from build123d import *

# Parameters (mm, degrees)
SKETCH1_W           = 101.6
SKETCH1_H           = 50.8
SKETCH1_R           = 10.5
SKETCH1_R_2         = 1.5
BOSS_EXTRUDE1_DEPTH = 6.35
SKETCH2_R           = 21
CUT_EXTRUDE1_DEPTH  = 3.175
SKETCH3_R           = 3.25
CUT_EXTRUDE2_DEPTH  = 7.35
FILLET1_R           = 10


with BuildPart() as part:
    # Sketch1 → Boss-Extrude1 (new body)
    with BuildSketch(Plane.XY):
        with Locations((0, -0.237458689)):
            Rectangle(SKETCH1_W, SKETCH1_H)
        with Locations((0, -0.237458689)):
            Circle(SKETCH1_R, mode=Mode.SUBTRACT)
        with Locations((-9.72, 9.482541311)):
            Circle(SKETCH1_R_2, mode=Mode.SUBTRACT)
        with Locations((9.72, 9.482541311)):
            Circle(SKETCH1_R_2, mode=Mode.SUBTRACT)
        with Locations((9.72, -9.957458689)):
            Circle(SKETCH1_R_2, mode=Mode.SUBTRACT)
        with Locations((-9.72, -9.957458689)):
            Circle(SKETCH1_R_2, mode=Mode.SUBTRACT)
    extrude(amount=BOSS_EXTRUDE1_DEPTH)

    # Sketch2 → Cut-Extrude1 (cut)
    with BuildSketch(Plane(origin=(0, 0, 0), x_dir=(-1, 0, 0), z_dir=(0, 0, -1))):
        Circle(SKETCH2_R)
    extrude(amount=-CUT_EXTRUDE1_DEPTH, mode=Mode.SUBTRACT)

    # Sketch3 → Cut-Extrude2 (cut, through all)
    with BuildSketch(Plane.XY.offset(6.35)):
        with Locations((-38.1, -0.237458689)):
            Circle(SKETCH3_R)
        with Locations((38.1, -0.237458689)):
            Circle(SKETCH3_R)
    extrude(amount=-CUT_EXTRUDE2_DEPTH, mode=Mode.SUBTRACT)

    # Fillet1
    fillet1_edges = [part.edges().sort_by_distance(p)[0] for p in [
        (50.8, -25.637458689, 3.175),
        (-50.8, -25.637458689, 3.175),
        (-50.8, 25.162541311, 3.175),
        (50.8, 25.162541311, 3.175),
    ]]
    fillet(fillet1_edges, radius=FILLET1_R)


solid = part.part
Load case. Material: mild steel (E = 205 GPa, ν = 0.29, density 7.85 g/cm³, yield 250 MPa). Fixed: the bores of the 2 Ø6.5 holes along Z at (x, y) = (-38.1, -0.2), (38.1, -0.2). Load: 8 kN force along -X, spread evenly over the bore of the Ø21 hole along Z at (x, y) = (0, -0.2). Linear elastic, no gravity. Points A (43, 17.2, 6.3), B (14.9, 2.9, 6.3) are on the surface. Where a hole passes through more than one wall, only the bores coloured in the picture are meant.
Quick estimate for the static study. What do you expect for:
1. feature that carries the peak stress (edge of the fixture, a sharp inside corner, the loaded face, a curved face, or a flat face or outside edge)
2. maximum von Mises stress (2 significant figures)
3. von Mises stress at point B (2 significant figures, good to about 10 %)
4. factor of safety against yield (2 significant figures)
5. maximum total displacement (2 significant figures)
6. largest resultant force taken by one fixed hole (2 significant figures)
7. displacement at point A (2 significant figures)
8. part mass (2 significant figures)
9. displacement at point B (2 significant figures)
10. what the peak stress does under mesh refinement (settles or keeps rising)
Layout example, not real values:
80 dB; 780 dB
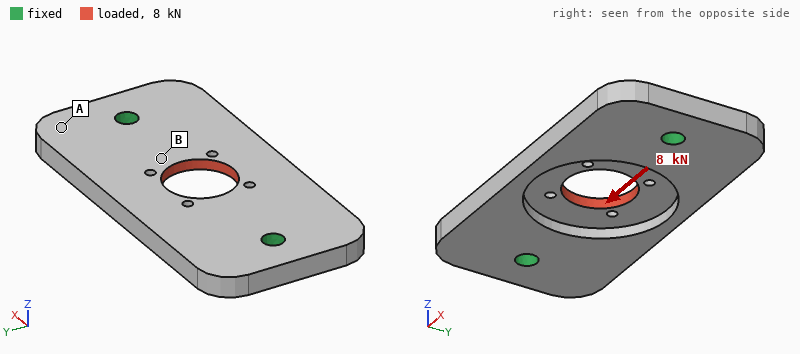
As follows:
a curved face; 170 MPa; 45 MPa; 1.5; 7.1 µm; 4.0 kN; 2.3 µm; 210 g; 5.3 µm; settles
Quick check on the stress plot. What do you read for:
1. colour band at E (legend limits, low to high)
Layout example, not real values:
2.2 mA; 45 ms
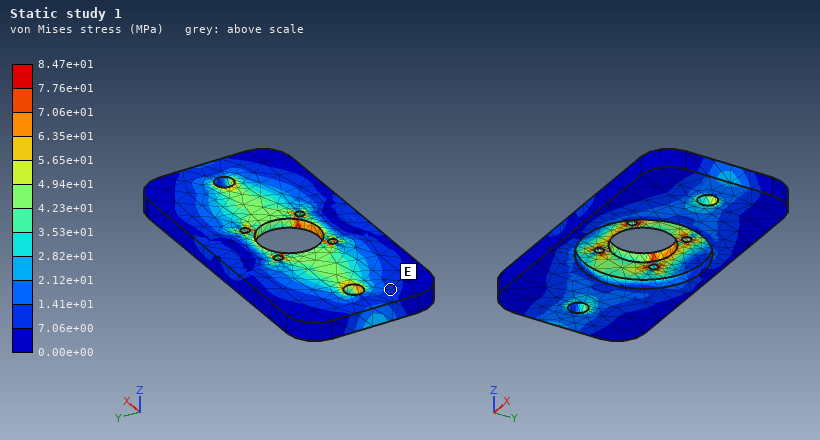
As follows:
7.06e+00 to 1.41e+01 MPa
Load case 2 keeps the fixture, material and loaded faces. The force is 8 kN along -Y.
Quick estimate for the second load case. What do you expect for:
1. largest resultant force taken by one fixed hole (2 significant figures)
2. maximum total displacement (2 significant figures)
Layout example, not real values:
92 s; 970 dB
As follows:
4.0 kN; 20 µm
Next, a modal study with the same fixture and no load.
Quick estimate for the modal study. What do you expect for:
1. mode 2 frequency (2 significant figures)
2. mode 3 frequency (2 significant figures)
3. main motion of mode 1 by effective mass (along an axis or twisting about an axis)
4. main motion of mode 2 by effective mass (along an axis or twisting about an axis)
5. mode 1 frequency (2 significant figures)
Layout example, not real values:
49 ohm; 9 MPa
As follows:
4900 Hz; 7700 Hz; twisting about X; along Z; 4600 Hz
